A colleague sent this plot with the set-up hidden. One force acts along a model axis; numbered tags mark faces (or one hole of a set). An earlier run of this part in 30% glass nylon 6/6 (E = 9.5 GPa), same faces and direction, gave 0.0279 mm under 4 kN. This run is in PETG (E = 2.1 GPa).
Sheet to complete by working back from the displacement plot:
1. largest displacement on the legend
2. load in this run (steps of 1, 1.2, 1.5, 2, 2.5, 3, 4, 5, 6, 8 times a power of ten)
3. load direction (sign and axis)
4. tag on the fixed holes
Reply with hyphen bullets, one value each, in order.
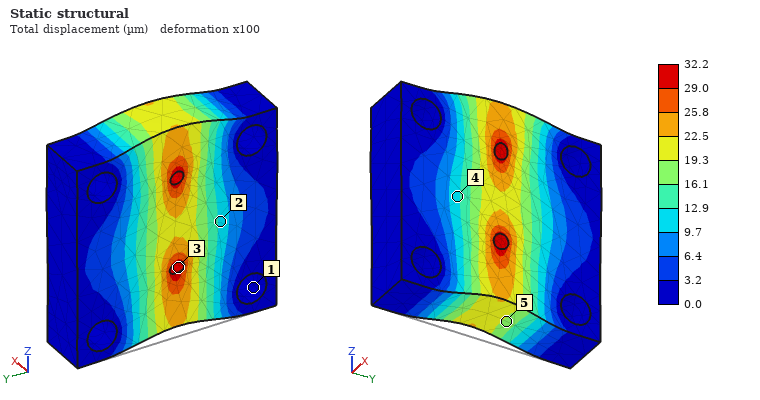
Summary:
- 32.2 µm
- 1 kN
- +Z
- 1
